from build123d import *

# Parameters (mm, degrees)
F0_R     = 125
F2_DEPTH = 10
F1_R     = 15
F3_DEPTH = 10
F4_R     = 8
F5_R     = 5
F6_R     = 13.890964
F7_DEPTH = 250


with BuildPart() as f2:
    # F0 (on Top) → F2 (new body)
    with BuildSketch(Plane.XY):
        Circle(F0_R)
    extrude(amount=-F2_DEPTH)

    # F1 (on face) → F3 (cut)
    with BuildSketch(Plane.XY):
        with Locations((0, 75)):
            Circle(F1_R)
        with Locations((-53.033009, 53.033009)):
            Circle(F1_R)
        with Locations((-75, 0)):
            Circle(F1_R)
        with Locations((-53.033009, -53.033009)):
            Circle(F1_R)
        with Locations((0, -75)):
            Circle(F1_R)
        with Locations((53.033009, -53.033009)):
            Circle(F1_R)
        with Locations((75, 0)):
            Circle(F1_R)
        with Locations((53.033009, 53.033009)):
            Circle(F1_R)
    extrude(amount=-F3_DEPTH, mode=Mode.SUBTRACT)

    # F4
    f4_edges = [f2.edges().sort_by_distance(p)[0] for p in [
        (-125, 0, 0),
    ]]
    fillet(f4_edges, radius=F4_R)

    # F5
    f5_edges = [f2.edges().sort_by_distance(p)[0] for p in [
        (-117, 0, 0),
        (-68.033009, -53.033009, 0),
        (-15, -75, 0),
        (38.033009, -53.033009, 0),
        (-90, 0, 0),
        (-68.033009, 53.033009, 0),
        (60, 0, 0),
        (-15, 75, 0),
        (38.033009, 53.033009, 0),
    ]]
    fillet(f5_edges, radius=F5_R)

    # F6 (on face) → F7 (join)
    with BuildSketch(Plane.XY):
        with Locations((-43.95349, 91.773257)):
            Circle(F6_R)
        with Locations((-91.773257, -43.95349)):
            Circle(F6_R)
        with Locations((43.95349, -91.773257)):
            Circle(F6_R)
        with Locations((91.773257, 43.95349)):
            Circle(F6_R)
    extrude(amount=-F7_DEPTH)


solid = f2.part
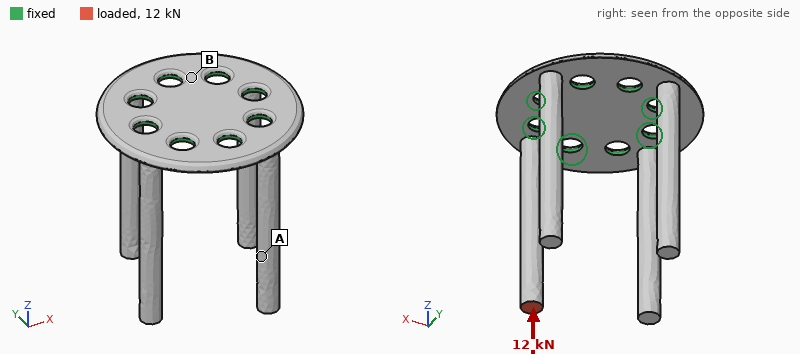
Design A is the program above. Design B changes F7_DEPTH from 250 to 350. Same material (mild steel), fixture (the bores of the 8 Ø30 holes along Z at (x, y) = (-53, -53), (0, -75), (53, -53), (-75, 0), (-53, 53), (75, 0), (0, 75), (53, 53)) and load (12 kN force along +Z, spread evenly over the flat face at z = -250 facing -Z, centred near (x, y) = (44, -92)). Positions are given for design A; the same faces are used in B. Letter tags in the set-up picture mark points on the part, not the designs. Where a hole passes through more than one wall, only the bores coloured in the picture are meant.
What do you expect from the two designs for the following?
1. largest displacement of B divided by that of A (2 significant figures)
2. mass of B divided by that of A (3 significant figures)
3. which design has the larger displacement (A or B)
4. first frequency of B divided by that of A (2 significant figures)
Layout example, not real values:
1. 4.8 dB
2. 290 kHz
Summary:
1. 1.4
2. 1.24
3. B
4. 0.55
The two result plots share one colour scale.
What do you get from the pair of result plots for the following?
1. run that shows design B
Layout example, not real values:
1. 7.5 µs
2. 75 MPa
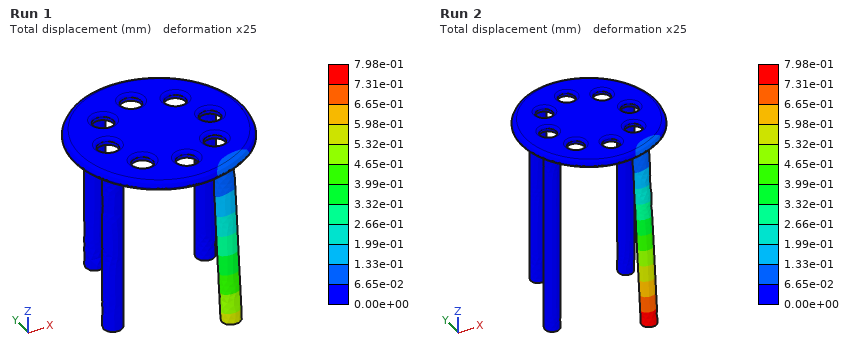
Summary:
1. Run 2
